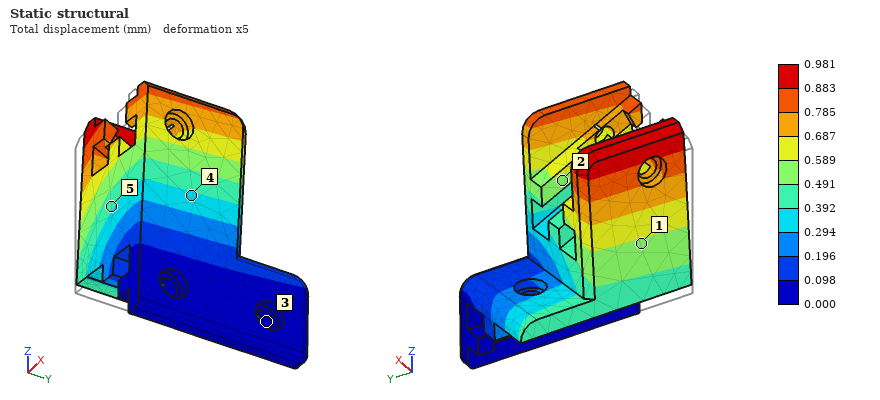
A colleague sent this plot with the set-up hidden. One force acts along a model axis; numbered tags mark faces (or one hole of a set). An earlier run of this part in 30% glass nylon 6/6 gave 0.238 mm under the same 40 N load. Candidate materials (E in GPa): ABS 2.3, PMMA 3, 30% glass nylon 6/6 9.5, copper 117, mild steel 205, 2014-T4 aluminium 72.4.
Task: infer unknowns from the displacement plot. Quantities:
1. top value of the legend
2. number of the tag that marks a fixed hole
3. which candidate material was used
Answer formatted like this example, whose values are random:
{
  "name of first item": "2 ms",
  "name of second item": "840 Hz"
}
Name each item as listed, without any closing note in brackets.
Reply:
{
  "top value of the legend": "0.981 mm",
  "number of the tag that marks a fixed hole": "3",
  "which candidate material was used": "ABS"
}
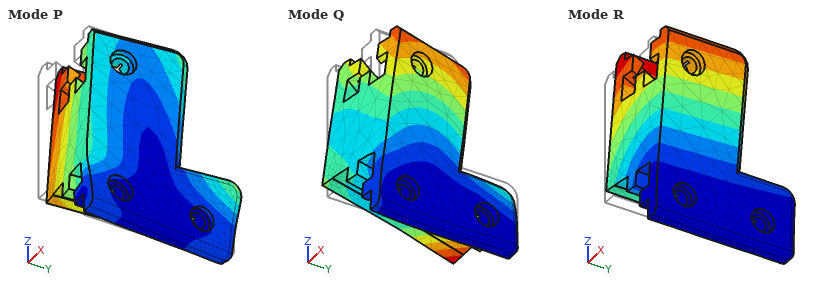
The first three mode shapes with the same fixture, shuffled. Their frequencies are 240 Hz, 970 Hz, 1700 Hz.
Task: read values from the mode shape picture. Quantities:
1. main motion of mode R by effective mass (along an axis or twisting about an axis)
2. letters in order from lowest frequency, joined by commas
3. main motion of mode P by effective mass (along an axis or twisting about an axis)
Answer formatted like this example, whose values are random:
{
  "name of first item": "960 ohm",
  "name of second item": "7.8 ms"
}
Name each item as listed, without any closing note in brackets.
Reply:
{
  "main motion of mode R by effective mass": "along X",
  "letters in order from lowest frequency, joined by commas": "R, P, Q",
  "main motion of mode P by effective mass": "along Y"
}
